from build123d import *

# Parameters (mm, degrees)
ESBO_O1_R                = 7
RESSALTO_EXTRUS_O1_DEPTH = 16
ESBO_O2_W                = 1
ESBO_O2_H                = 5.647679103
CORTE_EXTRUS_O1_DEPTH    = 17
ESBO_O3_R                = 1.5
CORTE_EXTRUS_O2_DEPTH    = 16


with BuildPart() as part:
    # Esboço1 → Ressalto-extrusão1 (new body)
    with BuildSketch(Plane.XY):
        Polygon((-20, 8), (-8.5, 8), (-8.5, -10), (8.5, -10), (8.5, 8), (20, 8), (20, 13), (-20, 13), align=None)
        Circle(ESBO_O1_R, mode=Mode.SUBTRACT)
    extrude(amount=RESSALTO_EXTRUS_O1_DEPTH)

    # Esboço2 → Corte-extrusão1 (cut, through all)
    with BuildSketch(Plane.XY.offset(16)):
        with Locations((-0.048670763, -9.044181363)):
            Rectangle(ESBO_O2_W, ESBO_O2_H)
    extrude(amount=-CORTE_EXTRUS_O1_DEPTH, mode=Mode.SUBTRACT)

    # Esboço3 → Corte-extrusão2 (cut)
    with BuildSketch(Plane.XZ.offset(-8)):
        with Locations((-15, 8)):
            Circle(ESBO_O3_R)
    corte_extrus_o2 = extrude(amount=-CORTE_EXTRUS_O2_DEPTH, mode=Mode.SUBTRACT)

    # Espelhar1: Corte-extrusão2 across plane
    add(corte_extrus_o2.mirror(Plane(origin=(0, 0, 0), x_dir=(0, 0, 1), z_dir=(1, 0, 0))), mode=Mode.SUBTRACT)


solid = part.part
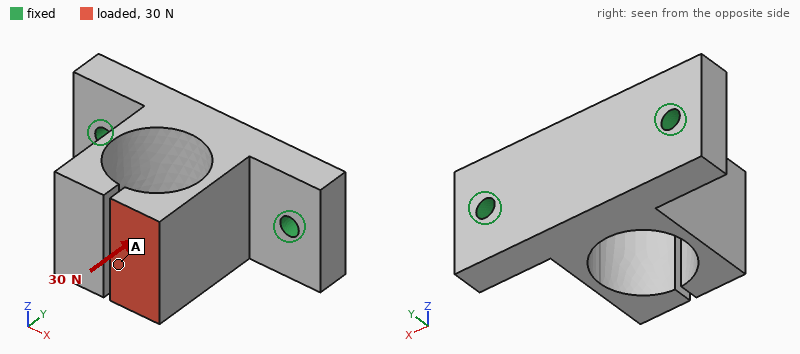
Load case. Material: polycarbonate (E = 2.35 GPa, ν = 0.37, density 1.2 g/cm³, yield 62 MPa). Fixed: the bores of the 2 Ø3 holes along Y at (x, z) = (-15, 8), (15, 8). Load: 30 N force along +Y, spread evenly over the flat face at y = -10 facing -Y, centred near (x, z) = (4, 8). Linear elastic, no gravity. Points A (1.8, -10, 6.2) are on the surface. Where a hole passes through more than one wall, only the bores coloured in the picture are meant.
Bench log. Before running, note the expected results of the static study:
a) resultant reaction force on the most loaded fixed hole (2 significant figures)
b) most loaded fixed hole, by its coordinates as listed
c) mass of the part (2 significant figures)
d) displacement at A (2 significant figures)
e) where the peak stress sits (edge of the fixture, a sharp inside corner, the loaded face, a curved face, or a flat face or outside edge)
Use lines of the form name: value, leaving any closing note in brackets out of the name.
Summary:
resultant reaction force on the most loaded fixed hole: 21 N
most loaded fixed hole, by its coordinates as listed: (15, 8)
mass of the part: 6.6 g
displacement at A: 0.53 mm
where the peak stress sits: a curved face
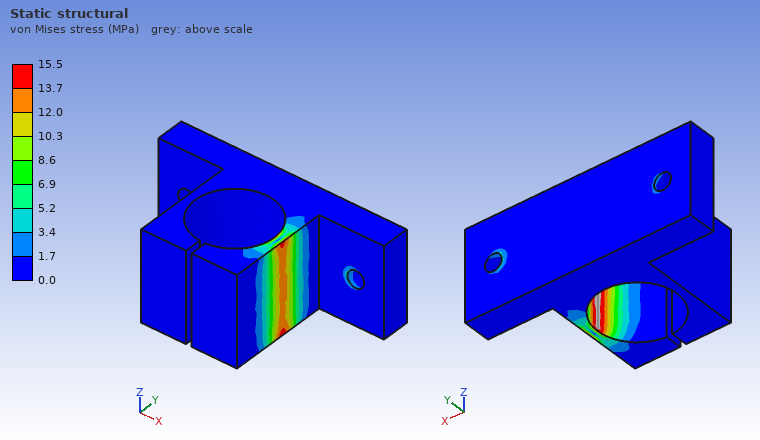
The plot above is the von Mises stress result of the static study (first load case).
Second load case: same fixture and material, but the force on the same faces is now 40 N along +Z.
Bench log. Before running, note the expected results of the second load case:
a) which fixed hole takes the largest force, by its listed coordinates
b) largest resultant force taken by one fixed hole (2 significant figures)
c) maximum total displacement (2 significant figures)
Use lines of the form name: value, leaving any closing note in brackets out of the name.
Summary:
which fixed hole takes the largest force, by its listed coordinates: (15, 8)
largest resultant force taken by one fixed hole: 26 N
maximum total displacement: 0.39 mm
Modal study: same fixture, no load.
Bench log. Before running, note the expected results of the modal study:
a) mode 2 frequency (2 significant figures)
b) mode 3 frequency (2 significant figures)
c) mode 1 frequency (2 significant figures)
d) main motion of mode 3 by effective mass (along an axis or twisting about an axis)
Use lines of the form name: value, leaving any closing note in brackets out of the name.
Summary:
mode 2 frequency: 960 Hz
mode 3 frequency: 1900 Hz
mode 1 frequency: 950 Hz
main motion of mode 3 by effective mass: along Z
